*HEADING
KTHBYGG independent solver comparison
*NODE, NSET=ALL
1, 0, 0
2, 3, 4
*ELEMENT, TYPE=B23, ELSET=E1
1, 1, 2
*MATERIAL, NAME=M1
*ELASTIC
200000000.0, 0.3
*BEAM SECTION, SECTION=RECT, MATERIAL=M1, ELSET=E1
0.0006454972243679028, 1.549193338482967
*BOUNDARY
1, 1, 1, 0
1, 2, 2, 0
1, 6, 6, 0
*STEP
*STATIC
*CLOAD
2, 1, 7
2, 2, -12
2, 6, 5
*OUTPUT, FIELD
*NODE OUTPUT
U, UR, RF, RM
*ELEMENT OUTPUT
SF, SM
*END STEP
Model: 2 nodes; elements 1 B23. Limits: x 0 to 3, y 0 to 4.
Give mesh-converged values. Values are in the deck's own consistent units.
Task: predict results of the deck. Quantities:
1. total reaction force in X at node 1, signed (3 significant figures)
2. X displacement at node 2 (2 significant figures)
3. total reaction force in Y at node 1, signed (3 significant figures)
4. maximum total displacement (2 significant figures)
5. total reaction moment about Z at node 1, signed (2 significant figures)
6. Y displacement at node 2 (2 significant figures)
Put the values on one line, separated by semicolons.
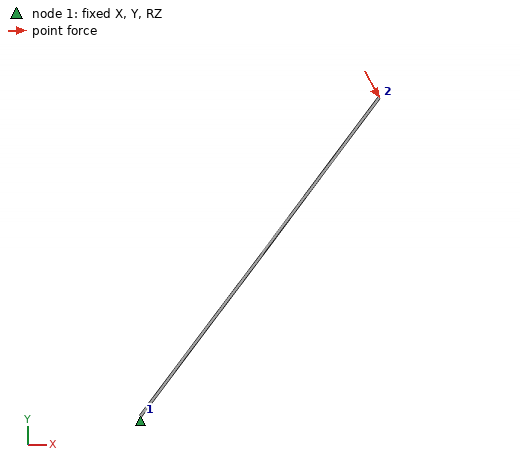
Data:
-7.00; 0.0093; 12.0; 0.012; 59; -0.0072
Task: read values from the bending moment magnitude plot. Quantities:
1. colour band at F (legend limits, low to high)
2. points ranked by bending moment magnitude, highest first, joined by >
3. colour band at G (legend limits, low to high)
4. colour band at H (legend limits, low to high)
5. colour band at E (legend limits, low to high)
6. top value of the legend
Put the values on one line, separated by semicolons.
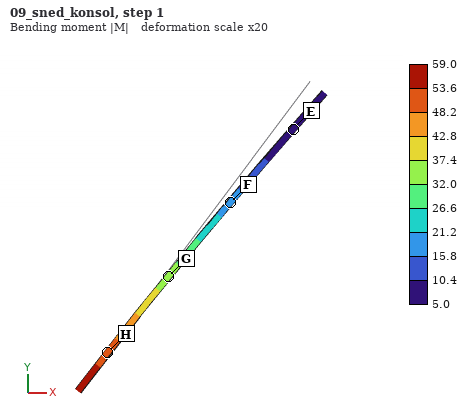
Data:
15.8 to 21.2; H > G > F > E; 32.0 to 37.4; 48.2 to 53.6; 5.0 to 10.4; 59.0
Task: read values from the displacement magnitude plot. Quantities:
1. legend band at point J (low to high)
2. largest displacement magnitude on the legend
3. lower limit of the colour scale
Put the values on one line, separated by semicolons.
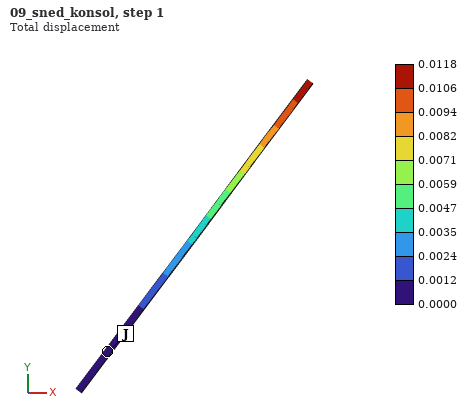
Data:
0.0000 to 0.0012; 0.0118; 0.0000
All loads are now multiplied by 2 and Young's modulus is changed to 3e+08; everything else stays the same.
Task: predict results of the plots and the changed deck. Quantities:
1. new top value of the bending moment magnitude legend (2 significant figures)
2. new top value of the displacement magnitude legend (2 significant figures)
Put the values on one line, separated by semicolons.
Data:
120; 0.016
